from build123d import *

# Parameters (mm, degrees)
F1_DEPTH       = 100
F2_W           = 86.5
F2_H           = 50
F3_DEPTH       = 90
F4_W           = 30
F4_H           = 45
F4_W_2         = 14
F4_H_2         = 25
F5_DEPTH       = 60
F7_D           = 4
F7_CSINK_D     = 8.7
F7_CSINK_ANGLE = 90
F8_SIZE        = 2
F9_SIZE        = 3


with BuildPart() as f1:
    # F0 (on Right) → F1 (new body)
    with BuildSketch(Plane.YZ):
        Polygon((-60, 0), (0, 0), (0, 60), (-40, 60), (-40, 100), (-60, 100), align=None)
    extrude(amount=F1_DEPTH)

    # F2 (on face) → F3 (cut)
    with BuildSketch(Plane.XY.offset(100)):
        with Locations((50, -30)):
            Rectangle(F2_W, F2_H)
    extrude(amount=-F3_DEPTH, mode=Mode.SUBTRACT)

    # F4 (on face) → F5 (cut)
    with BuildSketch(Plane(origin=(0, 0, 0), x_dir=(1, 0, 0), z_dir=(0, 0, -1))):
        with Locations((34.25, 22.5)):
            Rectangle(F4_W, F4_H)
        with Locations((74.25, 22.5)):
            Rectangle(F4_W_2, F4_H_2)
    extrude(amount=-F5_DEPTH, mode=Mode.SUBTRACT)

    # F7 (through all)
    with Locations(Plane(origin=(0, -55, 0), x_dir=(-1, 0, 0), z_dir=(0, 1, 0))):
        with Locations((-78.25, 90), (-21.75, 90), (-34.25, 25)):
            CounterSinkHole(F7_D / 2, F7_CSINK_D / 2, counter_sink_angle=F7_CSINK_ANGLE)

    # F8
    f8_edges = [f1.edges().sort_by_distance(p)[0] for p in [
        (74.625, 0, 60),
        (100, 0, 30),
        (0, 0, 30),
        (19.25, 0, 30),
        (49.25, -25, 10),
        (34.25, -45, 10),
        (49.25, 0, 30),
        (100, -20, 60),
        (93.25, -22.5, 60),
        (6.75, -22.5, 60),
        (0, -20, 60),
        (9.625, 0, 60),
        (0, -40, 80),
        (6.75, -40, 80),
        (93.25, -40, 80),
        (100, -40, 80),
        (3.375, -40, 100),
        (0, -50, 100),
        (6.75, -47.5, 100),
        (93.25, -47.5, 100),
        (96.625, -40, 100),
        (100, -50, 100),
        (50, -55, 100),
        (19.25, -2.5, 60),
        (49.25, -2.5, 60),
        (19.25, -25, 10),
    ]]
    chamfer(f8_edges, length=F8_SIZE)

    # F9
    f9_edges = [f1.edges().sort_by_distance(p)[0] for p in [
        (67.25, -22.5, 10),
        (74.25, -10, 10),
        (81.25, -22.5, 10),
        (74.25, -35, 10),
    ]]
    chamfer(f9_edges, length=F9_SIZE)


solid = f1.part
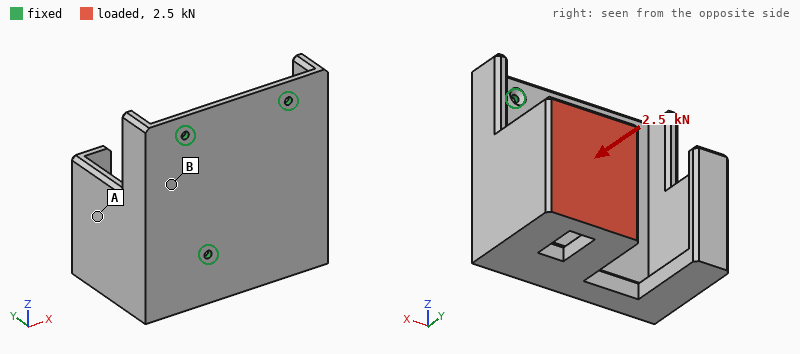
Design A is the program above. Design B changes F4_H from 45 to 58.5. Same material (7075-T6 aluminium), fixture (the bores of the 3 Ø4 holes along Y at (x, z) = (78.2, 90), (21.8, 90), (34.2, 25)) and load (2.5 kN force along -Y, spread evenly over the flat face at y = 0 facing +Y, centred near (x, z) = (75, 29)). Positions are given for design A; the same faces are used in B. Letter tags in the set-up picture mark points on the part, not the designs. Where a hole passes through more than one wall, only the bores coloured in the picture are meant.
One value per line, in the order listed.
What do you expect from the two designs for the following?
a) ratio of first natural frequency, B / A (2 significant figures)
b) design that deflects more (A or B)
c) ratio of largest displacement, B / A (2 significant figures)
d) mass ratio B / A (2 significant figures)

0.90
B
1.3
0.99
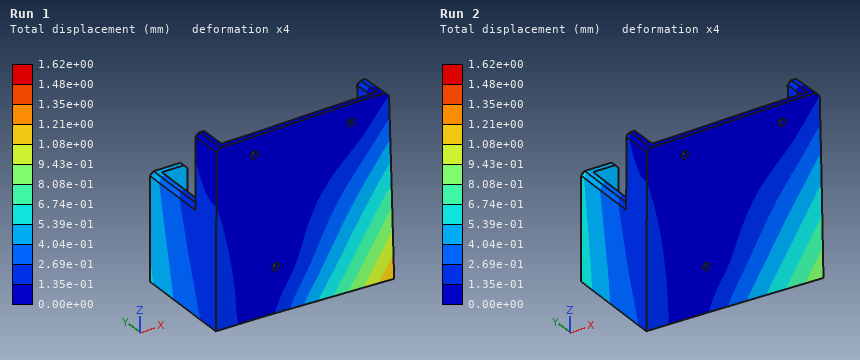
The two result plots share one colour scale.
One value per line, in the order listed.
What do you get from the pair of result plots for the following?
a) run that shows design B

Run 1
